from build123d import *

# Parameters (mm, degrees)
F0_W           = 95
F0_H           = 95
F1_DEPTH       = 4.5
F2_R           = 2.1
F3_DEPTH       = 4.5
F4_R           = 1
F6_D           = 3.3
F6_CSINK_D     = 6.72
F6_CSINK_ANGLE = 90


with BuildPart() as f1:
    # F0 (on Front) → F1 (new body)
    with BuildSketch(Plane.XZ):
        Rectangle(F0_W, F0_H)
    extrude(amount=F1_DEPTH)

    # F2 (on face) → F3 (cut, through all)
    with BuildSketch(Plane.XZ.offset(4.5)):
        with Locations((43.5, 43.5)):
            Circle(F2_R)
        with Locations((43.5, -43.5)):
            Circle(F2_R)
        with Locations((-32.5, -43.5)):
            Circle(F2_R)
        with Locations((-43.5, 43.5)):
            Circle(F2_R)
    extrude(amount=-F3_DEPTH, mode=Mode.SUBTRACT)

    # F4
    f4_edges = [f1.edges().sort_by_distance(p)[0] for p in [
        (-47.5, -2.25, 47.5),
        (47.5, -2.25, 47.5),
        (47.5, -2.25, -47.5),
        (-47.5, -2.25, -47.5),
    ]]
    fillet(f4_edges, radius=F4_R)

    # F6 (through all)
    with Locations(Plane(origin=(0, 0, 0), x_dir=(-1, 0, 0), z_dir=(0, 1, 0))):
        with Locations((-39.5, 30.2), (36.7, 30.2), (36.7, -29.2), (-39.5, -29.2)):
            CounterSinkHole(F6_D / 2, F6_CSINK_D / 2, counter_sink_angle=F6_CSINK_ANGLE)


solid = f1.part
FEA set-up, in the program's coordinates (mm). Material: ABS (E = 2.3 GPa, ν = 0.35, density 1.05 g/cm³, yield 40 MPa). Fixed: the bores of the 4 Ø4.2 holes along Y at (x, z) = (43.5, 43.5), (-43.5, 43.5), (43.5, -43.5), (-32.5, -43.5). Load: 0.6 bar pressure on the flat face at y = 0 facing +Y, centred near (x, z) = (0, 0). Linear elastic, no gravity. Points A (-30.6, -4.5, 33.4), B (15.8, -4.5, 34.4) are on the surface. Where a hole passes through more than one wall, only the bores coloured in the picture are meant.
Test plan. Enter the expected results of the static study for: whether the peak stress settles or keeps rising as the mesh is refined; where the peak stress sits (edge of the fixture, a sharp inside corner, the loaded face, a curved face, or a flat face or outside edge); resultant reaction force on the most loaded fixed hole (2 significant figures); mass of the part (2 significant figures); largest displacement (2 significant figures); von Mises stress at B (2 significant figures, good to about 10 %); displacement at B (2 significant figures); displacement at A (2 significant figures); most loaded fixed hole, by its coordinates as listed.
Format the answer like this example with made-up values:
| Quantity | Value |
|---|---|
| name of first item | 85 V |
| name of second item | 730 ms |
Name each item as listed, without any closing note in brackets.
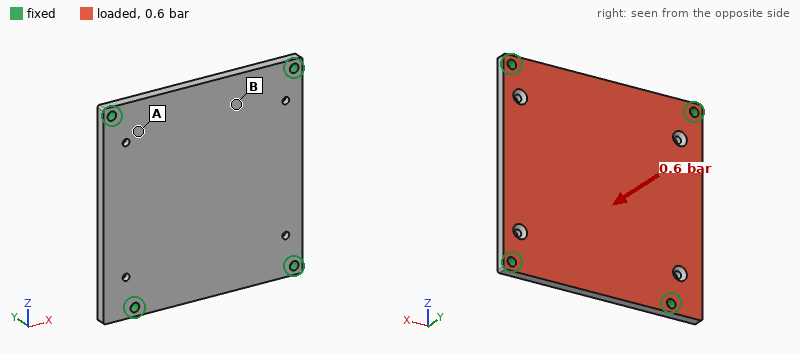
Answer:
| Quantity | Value |
|---|---|
| whether the peak stress settles or keeps rising as the mesh is refined | keeps rising |
| where the peak stress sits | edge of the fixture |
| resultant reaction force on the most loaded fixed hole | 160 N |
| mass of the part | 42 g |
| largest displacement | 1.4 mm |
| von Mises stress at B | 5.9 MPa |
| displacement at B | 0.84 mm |
| displacement at A | 0.47 mm |
| most loaded fixed hole, by its coordinates as listed | (-32.5, -43.5) |
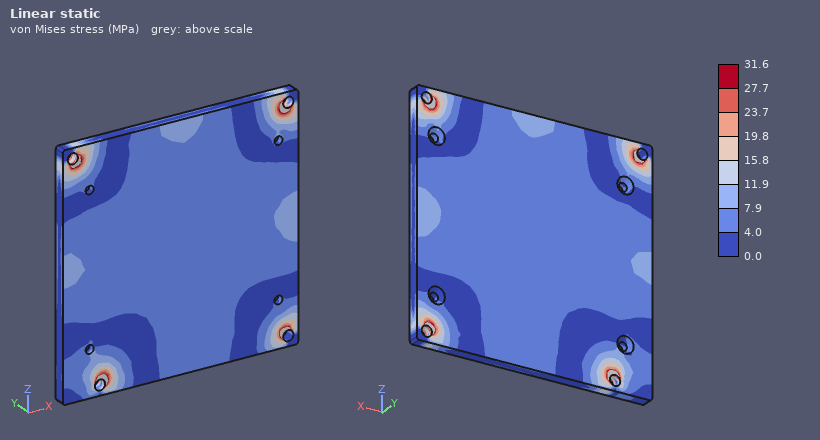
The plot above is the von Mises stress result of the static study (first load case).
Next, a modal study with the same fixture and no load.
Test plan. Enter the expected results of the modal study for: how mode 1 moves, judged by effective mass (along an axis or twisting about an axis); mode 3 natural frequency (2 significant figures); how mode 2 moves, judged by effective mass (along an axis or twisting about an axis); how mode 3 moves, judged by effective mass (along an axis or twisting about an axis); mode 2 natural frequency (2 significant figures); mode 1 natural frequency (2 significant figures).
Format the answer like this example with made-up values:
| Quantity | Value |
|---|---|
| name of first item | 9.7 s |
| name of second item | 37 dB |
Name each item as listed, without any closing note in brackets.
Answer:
| Quantity | Value |
|---|---|
| how mode 1 moves, judged by effective mass | along Y |
| mode 3 natural frequency | 1000 Hz |
| how mode 2 moves, judged by effective mass | twisting about Z |
| how mode 3 moves, judged by effective mass | twisting about X |
| mode 2 natural frequency | 950 Hz |
| mode 1 natural frequency | 580 Hz |
